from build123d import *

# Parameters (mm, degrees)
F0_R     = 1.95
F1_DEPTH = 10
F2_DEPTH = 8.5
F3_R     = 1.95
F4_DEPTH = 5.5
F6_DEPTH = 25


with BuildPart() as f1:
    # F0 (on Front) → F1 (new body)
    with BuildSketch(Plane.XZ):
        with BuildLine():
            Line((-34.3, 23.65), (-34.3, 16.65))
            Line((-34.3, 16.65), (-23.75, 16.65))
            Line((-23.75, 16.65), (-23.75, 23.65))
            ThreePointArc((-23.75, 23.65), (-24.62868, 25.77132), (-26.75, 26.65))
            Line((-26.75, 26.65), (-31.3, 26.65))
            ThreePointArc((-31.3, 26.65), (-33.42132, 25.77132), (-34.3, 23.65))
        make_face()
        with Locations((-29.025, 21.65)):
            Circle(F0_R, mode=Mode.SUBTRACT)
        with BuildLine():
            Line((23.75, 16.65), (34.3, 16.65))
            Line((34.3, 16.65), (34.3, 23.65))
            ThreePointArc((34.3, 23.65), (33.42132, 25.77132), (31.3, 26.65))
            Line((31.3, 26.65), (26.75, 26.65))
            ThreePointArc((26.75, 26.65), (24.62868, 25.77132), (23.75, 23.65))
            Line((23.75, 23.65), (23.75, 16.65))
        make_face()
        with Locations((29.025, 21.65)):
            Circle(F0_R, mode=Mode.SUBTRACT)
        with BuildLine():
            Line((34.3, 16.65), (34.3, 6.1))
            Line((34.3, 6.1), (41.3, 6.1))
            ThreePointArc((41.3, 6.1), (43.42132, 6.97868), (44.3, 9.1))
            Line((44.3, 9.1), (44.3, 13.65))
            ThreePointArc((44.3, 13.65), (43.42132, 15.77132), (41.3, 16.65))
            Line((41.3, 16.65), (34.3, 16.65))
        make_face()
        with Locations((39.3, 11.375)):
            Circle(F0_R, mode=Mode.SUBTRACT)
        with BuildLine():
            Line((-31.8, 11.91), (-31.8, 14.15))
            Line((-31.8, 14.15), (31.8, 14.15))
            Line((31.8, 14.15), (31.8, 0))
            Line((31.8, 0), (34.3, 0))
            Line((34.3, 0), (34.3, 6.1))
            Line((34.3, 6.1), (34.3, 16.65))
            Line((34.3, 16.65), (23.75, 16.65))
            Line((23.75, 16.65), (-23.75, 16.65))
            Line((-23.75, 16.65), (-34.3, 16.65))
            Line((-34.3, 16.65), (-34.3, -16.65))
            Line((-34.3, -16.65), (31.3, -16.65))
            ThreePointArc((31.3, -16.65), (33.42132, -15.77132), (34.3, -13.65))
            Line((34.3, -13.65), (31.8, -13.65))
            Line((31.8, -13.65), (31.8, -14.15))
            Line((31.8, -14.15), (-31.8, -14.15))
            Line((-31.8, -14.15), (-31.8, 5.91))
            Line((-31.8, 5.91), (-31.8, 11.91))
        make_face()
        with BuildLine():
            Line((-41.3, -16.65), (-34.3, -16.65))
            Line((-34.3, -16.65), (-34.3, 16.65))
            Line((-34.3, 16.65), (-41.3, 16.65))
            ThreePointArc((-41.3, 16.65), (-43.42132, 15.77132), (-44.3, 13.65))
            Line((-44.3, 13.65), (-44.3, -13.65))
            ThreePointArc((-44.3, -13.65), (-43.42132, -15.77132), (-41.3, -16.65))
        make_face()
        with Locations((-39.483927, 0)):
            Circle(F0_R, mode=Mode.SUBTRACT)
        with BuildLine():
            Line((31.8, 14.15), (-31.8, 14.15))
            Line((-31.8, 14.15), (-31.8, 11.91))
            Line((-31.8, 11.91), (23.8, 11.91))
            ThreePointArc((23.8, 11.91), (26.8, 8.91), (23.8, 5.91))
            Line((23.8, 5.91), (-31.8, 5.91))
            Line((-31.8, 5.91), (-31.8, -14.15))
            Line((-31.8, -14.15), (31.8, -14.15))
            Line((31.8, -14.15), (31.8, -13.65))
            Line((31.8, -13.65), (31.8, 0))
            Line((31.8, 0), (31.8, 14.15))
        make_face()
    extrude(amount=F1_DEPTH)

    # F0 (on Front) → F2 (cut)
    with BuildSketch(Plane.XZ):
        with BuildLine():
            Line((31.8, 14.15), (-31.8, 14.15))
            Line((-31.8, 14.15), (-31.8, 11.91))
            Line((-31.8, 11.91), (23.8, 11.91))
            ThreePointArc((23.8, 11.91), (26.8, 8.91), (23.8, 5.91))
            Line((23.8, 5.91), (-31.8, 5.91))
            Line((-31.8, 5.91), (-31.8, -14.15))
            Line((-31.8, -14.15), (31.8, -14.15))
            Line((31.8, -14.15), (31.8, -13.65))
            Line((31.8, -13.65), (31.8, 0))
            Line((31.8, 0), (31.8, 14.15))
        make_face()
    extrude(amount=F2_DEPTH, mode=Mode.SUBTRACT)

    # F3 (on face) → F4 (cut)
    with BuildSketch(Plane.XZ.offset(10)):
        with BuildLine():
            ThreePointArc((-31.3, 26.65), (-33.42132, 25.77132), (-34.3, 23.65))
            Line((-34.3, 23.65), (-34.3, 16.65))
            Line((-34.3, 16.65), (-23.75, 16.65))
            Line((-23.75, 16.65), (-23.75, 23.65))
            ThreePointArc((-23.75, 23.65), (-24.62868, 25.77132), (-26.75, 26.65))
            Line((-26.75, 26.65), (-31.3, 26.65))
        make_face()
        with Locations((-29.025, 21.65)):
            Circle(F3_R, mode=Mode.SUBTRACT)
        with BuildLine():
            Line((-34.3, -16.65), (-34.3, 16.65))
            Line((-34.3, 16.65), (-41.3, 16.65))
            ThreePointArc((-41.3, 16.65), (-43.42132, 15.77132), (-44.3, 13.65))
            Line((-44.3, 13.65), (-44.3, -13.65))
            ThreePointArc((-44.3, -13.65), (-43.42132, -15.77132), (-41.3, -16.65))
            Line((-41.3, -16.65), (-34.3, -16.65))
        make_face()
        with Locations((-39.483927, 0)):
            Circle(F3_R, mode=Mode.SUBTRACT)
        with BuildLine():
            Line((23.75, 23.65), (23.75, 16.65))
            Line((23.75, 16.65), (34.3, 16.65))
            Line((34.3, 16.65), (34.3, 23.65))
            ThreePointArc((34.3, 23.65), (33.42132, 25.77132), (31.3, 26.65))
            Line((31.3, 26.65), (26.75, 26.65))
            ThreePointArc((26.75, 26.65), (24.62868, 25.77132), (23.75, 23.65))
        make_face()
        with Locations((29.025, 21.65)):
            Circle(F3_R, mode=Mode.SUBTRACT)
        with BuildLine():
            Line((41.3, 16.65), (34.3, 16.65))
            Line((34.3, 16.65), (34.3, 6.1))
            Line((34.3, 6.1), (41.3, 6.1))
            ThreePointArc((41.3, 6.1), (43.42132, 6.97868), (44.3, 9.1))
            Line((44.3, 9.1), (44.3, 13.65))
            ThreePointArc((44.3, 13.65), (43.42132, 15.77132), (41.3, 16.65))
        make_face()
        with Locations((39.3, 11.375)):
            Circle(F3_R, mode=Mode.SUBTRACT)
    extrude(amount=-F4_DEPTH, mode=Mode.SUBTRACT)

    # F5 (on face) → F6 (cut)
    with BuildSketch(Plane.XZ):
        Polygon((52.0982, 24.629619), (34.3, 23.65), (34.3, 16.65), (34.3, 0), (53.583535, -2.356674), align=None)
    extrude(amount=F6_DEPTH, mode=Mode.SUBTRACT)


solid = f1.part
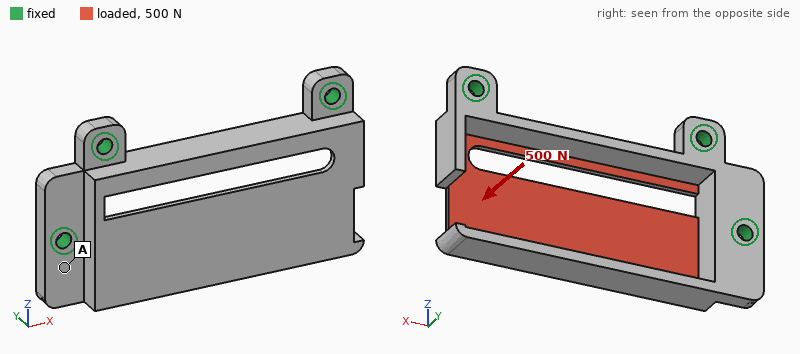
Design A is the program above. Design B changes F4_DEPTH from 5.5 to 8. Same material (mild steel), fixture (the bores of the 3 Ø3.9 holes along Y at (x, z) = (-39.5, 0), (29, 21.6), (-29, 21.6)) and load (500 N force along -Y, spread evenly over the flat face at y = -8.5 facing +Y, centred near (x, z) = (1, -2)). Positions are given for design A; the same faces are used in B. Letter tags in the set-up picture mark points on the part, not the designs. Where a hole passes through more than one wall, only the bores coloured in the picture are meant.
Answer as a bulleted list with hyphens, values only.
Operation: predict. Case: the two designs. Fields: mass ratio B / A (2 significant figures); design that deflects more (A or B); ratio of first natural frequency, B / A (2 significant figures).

- 0.86
- B
- 0.76
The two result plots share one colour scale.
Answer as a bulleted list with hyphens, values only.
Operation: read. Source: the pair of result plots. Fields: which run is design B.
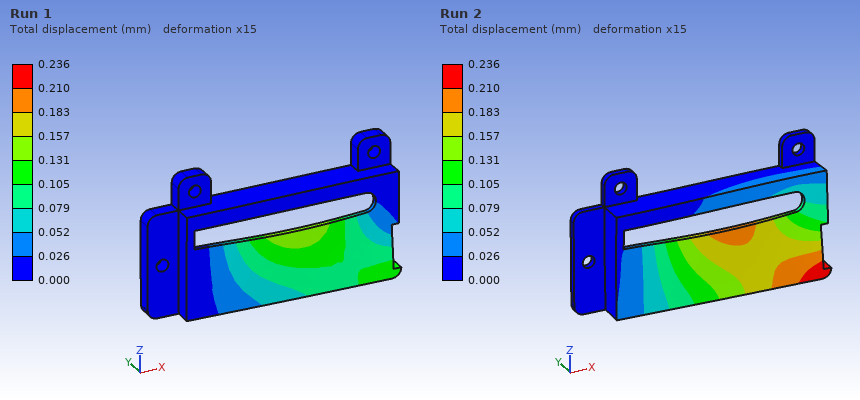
- Run 2
